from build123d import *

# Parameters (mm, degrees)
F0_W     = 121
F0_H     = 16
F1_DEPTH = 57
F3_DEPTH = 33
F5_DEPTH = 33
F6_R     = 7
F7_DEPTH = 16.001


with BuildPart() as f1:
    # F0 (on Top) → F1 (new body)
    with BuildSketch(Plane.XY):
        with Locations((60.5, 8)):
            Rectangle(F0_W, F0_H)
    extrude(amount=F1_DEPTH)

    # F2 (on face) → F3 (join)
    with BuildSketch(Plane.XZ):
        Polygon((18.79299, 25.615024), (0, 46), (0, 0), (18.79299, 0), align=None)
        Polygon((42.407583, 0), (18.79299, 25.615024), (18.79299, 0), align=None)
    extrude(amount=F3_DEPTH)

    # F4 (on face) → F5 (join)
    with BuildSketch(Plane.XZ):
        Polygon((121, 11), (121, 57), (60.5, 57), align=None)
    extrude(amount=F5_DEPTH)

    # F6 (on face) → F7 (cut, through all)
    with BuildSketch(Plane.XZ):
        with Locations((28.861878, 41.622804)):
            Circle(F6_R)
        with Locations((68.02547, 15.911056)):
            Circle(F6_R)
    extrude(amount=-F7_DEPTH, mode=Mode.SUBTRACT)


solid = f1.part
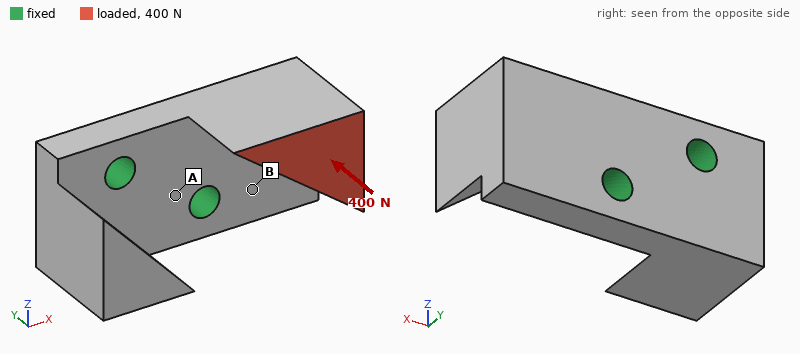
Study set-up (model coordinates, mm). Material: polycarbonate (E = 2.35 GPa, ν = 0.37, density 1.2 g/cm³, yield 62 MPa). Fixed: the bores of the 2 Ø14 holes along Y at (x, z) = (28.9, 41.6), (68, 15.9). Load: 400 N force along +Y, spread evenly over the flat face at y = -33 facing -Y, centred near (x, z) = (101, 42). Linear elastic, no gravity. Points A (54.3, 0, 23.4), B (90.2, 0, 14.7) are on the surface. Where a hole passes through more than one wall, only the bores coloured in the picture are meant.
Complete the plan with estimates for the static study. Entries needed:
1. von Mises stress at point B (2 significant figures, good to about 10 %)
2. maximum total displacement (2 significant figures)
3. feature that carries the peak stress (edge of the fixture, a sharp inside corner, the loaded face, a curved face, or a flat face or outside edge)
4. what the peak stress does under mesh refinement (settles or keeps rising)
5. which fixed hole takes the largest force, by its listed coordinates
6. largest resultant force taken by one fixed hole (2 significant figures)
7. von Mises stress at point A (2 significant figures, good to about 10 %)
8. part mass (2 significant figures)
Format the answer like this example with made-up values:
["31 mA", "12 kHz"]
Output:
["3.0 MPa", "0.46 mm", "edge of the fixture", "keeps rising", "(68, 15.9)", "430 N", "1.3 MPa", "220 g"]
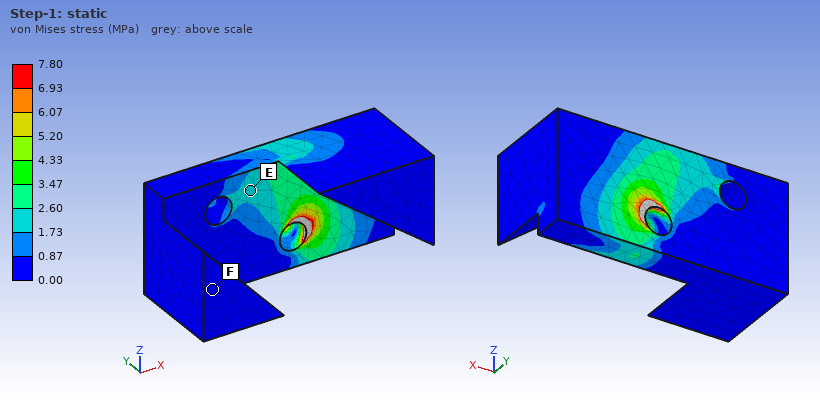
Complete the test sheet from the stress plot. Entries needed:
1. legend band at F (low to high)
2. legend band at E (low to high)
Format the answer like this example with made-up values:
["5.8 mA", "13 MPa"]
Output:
["0.00 to 0.87 MPa", "1.73 to 2.60 MPa"]
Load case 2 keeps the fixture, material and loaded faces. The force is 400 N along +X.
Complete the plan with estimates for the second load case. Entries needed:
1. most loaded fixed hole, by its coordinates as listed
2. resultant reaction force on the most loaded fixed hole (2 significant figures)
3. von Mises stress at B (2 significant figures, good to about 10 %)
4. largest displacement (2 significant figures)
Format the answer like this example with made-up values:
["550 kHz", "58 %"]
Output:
["(28.9, 41.6)", "310 N", "4.2 MPa", "0.59 mm"]
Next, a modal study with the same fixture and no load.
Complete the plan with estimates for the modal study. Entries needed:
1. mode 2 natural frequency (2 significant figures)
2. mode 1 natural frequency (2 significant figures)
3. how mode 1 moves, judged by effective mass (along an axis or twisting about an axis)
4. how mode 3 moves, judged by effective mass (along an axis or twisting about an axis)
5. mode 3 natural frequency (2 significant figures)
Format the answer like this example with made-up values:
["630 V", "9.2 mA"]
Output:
["970 Hz", "600 Hz", "along Y", "along Z", "1100 Hz"]
